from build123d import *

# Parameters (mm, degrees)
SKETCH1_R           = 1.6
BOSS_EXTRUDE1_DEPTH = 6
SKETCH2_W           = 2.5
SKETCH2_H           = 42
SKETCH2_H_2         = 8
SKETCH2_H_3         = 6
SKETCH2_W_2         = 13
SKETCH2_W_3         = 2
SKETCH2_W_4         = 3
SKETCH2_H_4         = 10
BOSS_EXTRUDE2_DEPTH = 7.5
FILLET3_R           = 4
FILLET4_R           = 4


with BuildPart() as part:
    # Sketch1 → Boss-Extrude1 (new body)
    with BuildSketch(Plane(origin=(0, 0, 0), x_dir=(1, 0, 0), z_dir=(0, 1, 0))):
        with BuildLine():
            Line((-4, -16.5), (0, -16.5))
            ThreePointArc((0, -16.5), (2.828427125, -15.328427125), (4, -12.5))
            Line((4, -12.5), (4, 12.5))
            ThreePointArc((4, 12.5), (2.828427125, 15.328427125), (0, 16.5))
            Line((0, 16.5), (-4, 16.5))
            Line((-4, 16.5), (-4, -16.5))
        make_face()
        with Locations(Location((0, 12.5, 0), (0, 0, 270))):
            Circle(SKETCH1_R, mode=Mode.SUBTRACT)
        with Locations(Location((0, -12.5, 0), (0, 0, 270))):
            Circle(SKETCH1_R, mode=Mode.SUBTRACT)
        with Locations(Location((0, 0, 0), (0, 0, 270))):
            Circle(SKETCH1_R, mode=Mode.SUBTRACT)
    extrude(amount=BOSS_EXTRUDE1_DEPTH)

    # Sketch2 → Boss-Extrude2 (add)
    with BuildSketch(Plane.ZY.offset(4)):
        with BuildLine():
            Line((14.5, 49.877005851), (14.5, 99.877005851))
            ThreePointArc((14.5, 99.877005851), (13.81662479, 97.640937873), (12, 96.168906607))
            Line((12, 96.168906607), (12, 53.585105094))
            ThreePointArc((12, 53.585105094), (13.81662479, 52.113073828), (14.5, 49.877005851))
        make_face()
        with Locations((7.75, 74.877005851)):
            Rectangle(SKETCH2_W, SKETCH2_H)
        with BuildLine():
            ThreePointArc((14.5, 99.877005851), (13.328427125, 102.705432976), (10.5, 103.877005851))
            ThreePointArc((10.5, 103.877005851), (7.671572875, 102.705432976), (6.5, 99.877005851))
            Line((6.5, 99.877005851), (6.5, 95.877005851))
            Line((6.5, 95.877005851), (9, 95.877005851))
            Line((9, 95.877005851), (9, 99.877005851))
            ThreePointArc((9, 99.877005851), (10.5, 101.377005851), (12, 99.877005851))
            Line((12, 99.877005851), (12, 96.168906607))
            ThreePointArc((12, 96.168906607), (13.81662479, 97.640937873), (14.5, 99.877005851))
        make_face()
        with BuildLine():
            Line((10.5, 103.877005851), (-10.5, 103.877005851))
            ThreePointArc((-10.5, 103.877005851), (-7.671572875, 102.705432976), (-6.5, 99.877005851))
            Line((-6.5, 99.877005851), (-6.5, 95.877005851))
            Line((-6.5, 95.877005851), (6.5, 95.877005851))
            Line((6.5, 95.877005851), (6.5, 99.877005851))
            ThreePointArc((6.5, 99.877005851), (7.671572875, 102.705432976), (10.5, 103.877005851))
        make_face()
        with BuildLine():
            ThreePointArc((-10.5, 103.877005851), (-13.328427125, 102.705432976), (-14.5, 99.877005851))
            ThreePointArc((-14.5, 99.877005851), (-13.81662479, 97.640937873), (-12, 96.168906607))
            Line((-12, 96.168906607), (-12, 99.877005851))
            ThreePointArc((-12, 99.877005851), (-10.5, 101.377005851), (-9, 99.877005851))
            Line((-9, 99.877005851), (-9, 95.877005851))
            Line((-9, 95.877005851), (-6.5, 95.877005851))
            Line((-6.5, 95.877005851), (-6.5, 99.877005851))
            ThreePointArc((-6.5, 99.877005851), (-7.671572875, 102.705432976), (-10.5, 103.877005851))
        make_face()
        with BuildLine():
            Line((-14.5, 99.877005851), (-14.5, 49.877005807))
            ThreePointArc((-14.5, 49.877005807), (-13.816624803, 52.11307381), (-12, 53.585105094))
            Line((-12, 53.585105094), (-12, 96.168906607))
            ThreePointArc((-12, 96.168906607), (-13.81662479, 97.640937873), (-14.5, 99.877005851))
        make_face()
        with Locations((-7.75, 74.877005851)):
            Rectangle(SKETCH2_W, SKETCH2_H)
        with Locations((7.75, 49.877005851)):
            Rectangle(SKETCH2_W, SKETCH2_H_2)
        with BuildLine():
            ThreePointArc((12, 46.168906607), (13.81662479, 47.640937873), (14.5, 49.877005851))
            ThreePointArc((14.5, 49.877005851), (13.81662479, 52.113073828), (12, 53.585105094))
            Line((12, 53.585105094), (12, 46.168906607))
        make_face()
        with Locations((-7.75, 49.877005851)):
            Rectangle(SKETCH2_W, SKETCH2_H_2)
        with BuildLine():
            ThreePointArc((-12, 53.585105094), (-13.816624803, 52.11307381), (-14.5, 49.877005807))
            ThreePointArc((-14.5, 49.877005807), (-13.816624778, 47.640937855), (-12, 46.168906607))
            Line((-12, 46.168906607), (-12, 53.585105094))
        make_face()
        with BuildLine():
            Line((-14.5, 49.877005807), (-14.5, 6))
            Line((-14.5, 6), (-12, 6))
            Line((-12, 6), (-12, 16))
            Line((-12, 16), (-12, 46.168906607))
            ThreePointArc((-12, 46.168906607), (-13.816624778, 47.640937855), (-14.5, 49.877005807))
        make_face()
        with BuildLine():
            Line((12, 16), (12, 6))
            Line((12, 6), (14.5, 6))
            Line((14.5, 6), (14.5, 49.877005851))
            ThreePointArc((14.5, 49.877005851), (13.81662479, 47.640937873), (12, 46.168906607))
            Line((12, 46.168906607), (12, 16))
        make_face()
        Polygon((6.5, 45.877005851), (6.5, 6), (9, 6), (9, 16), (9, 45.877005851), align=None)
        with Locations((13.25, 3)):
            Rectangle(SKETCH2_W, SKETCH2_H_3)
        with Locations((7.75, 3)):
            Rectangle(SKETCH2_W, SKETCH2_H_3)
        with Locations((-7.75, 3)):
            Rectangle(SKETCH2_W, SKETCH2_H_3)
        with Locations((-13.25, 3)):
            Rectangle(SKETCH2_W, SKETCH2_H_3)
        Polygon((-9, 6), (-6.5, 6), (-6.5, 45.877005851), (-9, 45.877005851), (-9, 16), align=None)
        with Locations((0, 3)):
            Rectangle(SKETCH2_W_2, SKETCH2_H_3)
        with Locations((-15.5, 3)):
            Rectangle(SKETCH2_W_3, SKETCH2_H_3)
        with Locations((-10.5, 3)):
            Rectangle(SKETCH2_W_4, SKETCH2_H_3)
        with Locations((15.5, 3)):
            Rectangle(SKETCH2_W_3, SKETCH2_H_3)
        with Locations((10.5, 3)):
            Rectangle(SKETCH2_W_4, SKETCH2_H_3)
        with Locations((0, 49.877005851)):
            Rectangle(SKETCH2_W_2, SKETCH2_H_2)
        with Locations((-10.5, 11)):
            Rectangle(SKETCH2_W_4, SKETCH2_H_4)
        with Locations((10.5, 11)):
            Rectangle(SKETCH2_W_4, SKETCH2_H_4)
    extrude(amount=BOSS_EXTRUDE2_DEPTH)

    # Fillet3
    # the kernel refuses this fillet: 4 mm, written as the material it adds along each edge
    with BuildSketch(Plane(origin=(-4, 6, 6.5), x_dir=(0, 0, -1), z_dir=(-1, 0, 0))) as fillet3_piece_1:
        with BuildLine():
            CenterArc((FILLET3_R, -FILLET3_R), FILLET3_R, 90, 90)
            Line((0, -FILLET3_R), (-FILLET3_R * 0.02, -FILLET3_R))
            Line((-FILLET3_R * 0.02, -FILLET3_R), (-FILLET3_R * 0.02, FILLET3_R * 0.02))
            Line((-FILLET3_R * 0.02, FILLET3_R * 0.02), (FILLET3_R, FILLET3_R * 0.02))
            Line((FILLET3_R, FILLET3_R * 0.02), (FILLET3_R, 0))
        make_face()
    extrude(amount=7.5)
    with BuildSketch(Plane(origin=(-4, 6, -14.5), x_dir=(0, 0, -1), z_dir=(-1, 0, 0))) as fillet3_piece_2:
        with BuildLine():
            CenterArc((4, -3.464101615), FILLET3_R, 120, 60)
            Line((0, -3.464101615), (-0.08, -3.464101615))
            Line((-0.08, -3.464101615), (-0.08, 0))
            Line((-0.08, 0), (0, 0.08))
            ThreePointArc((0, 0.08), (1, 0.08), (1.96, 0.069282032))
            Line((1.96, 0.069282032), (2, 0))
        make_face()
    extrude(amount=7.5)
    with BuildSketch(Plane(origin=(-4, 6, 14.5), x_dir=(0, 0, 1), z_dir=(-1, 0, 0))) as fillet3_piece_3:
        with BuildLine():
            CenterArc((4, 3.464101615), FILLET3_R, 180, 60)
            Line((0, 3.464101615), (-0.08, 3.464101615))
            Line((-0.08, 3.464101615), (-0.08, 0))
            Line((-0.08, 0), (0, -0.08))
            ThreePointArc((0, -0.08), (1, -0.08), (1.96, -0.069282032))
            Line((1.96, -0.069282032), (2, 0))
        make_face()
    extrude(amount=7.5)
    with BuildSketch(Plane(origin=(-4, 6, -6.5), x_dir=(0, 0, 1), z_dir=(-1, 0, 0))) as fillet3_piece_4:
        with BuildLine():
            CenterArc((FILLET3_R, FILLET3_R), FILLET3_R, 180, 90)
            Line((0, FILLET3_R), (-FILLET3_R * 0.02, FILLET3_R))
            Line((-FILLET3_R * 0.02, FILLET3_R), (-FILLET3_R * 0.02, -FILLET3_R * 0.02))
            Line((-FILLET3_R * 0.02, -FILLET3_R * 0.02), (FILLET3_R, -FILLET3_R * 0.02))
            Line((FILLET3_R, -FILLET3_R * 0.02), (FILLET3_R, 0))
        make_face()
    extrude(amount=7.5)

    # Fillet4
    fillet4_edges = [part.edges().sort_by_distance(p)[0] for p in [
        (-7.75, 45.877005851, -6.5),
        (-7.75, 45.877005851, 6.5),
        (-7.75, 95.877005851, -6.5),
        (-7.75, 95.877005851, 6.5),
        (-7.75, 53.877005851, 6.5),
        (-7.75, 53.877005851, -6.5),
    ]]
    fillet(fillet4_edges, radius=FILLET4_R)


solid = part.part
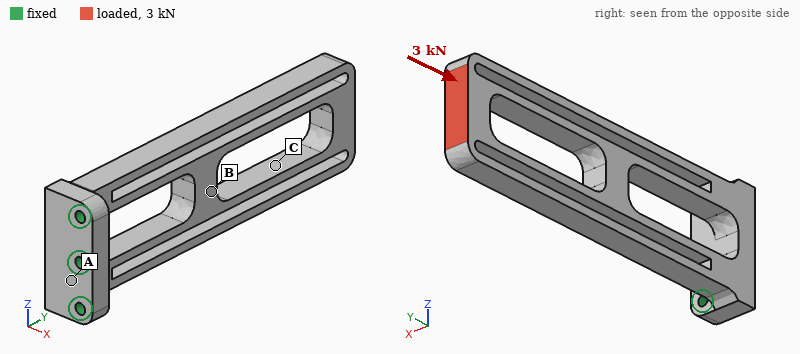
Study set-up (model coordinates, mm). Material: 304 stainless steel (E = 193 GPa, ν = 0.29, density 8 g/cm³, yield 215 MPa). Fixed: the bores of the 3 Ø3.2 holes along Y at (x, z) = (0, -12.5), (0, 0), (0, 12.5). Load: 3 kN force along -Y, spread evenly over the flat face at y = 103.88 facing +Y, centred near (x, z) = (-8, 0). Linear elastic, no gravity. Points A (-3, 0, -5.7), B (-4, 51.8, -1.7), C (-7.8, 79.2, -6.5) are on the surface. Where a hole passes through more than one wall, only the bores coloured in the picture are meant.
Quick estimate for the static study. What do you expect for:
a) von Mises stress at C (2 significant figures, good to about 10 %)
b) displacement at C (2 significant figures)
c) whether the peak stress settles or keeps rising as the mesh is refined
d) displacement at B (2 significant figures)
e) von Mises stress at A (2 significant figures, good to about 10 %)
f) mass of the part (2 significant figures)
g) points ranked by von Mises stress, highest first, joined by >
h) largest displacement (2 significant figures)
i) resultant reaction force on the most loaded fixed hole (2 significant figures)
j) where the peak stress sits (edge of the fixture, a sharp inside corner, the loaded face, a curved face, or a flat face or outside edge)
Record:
65 MPa
73 µm
keeps rising
45 µm
38 MPa
100 g
C > A > B
98 µm
1.0 kN
edge of the fixture
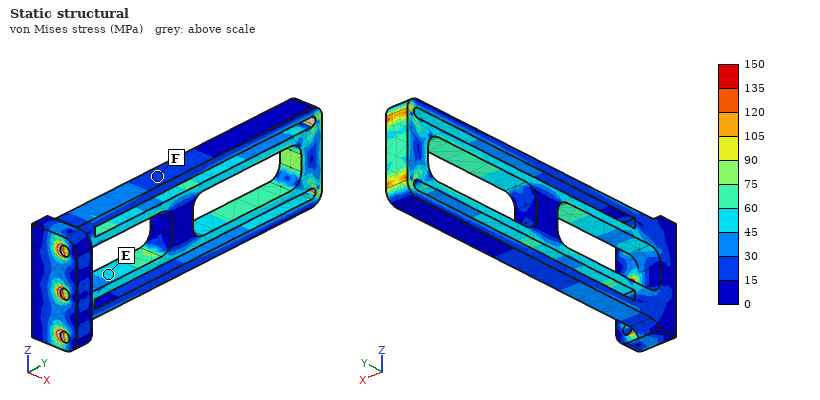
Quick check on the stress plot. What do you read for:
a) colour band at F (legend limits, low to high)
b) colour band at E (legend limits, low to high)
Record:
15 to 30 MPa
45 to 60 MPa
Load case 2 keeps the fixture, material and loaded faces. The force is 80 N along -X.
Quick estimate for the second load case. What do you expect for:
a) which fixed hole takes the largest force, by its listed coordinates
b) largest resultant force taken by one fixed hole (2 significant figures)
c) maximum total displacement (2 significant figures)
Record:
(0, 0)
88 N
0.38 mm
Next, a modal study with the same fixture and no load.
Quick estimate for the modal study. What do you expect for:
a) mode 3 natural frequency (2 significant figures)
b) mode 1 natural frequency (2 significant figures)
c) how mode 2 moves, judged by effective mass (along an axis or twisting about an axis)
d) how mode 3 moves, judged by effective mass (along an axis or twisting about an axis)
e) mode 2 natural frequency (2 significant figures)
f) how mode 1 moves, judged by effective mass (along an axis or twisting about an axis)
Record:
1500 Hz
490 Hz
along Z
twisting about Y
650 Hz
along X
